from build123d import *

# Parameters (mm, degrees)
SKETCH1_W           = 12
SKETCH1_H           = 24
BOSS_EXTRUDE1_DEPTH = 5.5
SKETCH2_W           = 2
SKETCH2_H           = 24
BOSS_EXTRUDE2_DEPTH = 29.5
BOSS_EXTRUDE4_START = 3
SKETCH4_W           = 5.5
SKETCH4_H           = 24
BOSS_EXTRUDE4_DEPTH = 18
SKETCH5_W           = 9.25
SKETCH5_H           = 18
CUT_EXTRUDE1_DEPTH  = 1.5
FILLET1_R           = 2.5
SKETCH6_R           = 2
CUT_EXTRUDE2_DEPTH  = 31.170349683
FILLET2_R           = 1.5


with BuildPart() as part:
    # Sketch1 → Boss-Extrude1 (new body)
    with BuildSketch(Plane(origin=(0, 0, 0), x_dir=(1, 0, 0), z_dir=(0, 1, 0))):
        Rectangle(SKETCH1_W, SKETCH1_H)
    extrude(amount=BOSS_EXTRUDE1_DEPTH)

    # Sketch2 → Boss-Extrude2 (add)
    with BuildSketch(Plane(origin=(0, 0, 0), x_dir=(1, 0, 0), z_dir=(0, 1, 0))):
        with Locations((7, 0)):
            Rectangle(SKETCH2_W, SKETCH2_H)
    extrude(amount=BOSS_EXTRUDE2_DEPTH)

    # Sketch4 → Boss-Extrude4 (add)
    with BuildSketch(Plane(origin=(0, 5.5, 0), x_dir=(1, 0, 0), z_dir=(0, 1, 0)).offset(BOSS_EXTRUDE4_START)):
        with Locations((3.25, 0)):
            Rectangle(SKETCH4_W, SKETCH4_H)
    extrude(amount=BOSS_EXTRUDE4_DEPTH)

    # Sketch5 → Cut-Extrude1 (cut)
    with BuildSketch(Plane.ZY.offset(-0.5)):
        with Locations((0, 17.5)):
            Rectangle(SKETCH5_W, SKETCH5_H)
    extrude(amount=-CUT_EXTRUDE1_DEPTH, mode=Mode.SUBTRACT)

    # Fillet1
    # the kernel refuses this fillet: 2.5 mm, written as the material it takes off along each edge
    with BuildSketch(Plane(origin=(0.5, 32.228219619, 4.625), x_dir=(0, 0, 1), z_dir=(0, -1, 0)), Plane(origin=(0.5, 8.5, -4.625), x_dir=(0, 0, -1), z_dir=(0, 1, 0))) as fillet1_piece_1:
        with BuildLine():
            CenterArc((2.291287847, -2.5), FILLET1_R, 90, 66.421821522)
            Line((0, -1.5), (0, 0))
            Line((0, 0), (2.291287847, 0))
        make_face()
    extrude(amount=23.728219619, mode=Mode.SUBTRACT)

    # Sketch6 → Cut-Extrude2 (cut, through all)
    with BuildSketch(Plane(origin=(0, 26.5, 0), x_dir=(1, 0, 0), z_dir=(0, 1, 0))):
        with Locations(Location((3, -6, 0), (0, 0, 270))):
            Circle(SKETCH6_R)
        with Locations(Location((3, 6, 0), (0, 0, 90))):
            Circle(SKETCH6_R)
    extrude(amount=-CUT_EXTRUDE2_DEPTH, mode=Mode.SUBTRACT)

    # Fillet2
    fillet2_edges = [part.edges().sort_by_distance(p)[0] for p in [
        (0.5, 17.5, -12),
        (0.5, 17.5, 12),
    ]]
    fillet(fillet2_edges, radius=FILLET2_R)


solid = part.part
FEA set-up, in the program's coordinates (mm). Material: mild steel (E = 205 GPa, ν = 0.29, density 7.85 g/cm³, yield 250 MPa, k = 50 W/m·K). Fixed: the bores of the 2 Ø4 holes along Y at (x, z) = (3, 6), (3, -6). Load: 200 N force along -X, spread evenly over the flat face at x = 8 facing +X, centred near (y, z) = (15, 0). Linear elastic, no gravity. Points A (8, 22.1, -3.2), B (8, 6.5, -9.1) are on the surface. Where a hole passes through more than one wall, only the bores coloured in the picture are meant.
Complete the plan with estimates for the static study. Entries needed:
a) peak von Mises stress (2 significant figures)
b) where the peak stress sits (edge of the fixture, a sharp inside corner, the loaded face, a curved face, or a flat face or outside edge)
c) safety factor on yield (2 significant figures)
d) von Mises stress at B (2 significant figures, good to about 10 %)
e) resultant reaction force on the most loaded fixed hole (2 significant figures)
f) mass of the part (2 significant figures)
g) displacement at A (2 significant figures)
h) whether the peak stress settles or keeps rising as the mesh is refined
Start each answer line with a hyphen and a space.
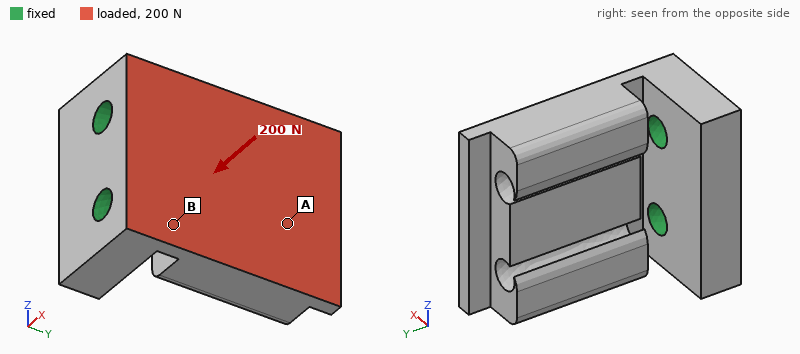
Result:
- 110 MPa
- the loaded face
- 2.3
- 97 MPa
- 100 N
- 35 g
- 41 µm
- settles
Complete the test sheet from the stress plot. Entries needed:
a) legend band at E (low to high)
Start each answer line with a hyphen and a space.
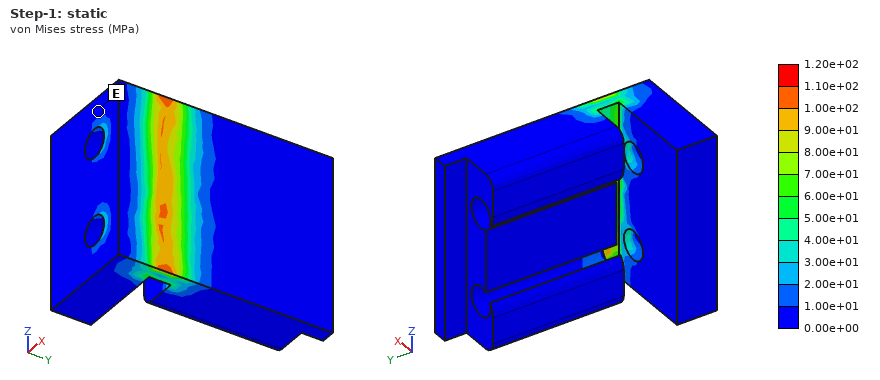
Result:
- 0.00e+00 to 1.00e+01 MPa
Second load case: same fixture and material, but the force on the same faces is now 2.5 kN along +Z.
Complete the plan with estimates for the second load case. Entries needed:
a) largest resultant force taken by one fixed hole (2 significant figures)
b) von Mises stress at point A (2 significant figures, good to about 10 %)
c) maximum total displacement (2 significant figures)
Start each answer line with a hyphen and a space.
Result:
- 2.2 kN
- 45 MPa
- 31 µm
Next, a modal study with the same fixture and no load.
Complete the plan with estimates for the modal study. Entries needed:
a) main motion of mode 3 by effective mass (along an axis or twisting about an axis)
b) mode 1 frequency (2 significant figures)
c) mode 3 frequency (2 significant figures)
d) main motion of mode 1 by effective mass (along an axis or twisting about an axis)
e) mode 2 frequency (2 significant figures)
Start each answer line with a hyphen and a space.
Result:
- along Z
- 2200 Hz
- 12 kHz
- along X
- 8900 Hz
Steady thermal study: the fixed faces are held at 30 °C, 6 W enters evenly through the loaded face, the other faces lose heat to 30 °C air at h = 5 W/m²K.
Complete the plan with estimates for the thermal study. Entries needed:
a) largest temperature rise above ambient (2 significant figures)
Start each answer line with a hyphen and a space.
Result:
- 19 K
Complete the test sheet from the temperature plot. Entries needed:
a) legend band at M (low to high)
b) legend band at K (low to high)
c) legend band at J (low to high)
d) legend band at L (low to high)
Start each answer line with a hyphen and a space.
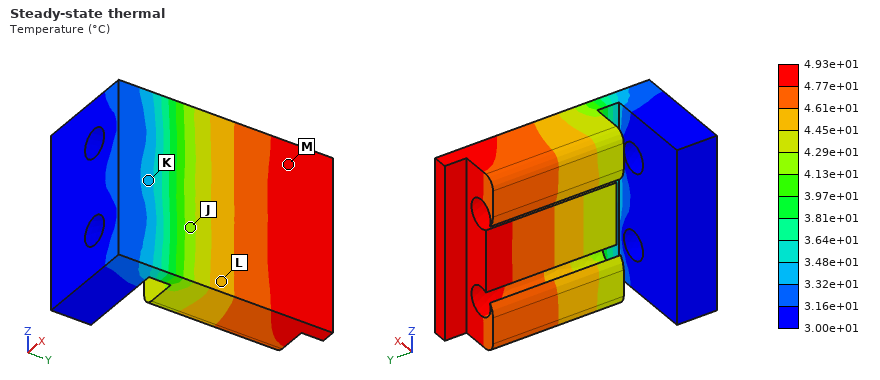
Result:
- 4.77e+01 to 4.93e+01 °C
- 3.32e+01 to 3.48e+01 °C
- 4.13e+01 to 4.29e+01 °C
- 4.45e+01 to 4.61e+01 °C
